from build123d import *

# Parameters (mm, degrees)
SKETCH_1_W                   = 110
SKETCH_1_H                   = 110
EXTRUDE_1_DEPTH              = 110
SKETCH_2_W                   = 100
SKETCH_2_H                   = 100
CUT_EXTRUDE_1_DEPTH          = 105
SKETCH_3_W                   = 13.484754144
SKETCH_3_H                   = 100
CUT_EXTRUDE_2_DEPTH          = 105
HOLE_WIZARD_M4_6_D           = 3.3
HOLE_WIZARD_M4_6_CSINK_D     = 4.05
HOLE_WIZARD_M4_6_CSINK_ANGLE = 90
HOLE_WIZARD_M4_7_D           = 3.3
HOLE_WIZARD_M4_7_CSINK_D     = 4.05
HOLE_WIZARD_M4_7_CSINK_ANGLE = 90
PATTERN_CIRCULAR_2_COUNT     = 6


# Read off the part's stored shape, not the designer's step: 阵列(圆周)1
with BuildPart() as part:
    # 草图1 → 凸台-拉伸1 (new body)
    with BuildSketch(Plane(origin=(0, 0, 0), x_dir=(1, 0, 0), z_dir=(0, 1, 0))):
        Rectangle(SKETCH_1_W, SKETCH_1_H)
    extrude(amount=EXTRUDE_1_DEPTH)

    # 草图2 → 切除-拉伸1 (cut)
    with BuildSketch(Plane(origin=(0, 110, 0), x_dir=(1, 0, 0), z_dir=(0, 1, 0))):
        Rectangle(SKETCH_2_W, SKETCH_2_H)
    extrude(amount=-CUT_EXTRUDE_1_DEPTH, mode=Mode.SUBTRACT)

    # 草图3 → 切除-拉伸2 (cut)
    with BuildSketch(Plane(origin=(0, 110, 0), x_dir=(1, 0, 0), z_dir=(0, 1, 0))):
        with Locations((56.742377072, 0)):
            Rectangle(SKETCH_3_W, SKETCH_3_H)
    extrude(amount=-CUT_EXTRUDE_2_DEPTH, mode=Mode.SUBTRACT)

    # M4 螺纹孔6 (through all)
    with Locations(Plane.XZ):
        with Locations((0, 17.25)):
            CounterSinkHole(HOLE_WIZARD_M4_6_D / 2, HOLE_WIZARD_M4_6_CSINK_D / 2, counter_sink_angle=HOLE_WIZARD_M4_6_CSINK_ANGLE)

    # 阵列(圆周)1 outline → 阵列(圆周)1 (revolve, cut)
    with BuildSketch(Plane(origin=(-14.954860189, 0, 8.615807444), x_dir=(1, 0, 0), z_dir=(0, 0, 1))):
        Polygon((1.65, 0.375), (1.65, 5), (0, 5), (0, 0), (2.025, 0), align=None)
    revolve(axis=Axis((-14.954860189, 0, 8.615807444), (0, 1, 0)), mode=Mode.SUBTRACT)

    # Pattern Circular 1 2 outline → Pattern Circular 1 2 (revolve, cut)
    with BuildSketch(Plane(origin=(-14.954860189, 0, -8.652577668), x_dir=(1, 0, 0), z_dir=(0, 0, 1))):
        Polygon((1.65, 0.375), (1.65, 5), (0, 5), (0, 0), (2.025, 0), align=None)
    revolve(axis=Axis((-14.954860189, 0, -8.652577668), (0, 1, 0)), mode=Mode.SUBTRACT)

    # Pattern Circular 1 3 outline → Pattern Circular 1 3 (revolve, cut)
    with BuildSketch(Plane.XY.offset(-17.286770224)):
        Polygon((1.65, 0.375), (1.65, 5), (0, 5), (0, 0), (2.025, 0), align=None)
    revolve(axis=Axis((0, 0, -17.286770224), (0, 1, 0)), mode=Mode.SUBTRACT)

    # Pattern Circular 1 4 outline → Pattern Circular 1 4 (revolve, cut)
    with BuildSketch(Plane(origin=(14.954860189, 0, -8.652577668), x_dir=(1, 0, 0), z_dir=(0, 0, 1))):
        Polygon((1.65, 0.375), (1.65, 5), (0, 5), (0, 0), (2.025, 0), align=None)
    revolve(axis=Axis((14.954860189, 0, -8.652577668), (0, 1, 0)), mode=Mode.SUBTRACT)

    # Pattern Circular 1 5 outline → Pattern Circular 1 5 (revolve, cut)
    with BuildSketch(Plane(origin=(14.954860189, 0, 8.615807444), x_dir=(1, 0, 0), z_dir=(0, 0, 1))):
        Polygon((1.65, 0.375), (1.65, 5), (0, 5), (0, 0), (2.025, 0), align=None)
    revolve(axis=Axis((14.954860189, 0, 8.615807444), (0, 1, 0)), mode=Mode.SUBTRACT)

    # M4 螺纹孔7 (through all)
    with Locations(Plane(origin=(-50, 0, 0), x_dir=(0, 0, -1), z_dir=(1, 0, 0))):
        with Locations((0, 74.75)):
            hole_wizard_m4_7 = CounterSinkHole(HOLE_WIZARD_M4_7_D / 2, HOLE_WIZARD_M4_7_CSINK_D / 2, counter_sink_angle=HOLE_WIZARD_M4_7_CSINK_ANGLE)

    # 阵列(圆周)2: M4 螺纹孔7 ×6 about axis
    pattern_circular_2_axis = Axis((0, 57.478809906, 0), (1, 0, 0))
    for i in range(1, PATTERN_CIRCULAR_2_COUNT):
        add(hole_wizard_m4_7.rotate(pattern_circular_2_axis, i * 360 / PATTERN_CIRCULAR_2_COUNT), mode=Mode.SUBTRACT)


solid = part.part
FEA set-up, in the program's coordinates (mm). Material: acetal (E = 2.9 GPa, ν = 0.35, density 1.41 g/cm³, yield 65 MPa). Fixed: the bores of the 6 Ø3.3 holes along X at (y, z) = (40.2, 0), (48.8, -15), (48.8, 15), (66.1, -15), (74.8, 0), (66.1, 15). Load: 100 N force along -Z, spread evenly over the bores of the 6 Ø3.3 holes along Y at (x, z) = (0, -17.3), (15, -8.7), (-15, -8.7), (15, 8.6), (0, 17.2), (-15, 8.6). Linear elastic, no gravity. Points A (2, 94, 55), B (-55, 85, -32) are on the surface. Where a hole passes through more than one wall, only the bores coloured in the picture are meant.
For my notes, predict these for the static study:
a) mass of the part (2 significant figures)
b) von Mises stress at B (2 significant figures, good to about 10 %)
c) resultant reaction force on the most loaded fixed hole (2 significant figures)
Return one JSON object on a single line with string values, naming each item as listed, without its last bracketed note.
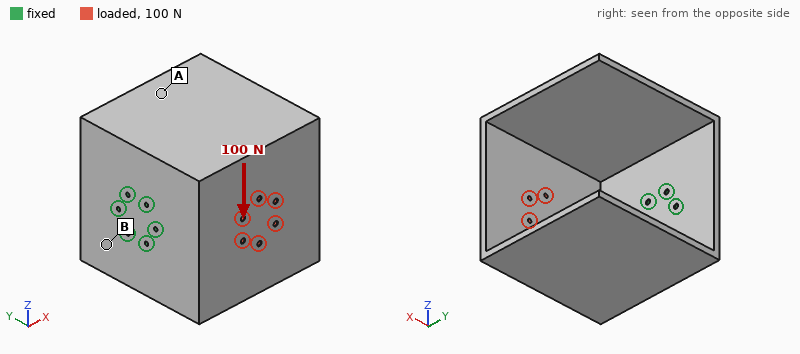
{"mass of the part": "320 g", "von Mises stress at B": "2.7 MPa", "resultant reaction force on the most loaded fixed hole": "110 N"}
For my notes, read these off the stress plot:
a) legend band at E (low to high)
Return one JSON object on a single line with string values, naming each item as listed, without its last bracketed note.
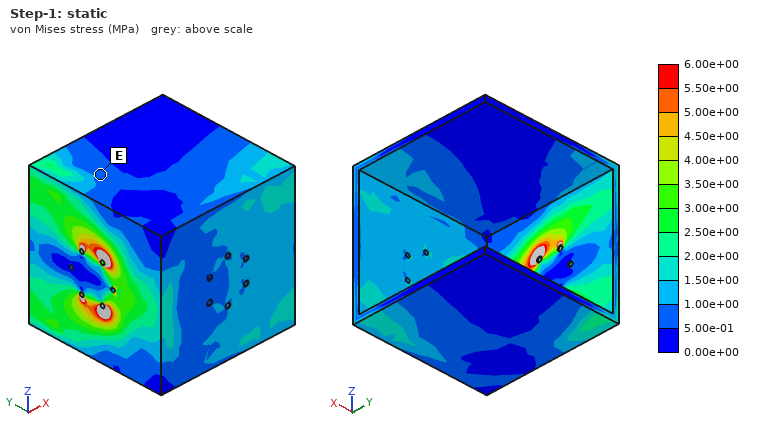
{"legend band at E": "5.00e-01 to 1.00e+00 MPa"}
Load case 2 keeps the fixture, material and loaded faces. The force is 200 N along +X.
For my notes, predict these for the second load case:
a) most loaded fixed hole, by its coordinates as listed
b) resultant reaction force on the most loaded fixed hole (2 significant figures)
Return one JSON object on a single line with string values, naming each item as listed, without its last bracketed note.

{"most loaded fixed hole, by its coordinates as listed": "(40.2, 0)", "resultant reaction force on the most loaded fixed hole": "190 N"}
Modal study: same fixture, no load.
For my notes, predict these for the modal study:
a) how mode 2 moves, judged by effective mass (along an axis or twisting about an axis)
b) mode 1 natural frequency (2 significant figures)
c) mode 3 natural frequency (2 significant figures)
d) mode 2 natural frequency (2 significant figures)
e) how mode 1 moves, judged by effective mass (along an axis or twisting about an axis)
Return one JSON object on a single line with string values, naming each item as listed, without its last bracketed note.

{"how mode 2 moves, judged by effective mass": "along Y", "mode 1 natural frequency": "77 Hz", "mode 3 natural frequency": "160 Hz", "mode 2 natural frequency": "96 Hz", "how mode 1 moves, judged by effective mass": "along Z"}
